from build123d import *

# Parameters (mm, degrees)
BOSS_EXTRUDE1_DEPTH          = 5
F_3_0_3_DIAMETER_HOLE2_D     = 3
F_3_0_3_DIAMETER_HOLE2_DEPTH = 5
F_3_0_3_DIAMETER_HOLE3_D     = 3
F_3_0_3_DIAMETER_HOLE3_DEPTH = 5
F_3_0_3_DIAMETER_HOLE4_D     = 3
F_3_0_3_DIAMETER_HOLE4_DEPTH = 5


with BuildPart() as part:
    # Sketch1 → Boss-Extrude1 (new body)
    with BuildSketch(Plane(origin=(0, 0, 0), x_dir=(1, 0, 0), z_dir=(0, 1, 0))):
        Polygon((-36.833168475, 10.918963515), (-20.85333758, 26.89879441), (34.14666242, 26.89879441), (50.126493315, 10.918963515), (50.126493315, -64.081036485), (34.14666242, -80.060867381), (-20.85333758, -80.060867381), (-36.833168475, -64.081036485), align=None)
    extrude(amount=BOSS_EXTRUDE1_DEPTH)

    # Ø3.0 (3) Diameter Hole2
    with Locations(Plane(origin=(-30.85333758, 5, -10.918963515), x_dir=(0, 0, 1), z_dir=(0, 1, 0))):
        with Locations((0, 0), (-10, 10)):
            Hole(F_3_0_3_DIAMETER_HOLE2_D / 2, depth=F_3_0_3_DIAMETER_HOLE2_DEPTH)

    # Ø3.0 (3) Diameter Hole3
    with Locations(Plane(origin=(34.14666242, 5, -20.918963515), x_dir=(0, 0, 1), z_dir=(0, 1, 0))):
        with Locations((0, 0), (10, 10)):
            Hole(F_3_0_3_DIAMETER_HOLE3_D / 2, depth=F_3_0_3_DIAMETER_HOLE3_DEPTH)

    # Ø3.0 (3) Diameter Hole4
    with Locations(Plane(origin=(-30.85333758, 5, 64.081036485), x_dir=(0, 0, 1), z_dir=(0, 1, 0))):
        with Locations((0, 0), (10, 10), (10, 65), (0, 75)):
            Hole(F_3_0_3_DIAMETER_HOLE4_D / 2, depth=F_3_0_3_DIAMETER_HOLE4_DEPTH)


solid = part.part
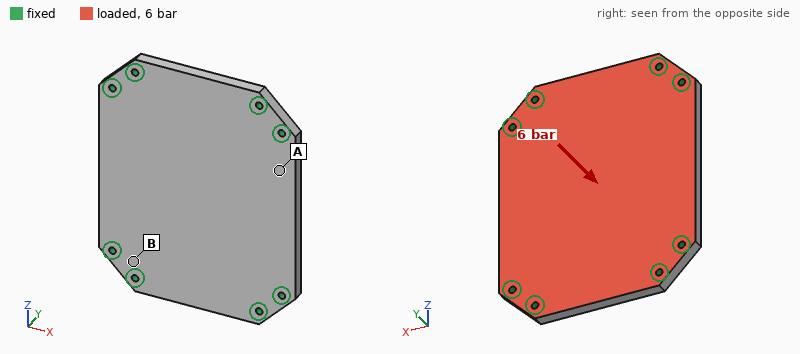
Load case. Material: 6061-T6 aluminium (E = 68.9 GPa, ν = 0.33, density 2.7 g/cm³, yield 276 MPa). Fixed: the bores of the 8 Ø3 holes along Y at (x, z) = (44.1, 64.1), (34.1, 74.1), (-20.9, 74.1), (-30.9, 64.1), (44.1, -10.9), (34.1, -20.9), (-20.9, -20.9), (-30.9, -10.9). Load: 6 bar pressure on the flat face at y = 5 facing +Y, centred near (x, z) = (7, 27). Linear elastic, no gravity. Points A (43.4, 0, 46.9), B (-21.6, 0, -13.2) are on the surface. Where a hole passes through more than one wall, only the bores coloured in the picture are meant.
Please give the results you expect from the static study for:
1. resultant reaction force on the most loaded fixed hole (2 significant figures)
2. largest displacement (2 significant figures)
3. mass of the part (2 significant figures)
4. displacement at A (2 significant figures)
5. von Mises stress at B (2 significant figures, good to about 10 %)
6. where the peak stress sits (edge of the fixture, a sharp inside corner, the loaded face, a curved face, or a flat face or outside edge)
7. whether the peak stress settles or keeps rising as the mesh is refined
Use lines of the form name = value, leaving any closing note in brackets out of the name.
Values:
resultant reaction force on the most loaded fixed hole = 840 N
largest displacement = 0.18 mm
mass of the part = 120 g
displacement at A = 0.066 mm
von Mises stress at B = 55 MPa
where the peak stress sits = edge of the fixture
whether the peak stress settles or keeps rising as the mesh is refined = keeps rising
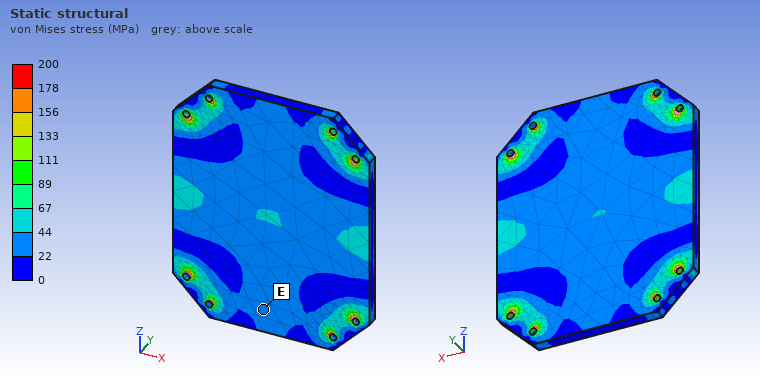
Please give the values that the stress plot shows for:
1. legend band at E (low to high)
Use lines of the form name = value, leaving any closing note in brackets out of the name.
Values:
legend band at E = 22 to 44 MPa
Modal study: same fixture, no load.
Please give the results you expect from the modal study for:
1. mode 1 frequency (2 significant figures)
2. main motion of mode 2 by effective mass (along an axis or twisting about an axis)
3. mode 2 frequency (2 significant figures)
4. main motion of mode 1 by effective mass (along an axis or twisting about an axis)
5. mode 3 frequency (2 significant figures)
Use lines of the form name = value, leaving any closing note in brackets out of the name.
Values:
mode 1 frequency = 3100 Hz
main motion of mode 2 by effective mass = twisting about Z
mode 2 frequency = 4800 Hz
main motion of mode 1 by effective mass = along Y
mode 3 frequency = 6400 Hz
